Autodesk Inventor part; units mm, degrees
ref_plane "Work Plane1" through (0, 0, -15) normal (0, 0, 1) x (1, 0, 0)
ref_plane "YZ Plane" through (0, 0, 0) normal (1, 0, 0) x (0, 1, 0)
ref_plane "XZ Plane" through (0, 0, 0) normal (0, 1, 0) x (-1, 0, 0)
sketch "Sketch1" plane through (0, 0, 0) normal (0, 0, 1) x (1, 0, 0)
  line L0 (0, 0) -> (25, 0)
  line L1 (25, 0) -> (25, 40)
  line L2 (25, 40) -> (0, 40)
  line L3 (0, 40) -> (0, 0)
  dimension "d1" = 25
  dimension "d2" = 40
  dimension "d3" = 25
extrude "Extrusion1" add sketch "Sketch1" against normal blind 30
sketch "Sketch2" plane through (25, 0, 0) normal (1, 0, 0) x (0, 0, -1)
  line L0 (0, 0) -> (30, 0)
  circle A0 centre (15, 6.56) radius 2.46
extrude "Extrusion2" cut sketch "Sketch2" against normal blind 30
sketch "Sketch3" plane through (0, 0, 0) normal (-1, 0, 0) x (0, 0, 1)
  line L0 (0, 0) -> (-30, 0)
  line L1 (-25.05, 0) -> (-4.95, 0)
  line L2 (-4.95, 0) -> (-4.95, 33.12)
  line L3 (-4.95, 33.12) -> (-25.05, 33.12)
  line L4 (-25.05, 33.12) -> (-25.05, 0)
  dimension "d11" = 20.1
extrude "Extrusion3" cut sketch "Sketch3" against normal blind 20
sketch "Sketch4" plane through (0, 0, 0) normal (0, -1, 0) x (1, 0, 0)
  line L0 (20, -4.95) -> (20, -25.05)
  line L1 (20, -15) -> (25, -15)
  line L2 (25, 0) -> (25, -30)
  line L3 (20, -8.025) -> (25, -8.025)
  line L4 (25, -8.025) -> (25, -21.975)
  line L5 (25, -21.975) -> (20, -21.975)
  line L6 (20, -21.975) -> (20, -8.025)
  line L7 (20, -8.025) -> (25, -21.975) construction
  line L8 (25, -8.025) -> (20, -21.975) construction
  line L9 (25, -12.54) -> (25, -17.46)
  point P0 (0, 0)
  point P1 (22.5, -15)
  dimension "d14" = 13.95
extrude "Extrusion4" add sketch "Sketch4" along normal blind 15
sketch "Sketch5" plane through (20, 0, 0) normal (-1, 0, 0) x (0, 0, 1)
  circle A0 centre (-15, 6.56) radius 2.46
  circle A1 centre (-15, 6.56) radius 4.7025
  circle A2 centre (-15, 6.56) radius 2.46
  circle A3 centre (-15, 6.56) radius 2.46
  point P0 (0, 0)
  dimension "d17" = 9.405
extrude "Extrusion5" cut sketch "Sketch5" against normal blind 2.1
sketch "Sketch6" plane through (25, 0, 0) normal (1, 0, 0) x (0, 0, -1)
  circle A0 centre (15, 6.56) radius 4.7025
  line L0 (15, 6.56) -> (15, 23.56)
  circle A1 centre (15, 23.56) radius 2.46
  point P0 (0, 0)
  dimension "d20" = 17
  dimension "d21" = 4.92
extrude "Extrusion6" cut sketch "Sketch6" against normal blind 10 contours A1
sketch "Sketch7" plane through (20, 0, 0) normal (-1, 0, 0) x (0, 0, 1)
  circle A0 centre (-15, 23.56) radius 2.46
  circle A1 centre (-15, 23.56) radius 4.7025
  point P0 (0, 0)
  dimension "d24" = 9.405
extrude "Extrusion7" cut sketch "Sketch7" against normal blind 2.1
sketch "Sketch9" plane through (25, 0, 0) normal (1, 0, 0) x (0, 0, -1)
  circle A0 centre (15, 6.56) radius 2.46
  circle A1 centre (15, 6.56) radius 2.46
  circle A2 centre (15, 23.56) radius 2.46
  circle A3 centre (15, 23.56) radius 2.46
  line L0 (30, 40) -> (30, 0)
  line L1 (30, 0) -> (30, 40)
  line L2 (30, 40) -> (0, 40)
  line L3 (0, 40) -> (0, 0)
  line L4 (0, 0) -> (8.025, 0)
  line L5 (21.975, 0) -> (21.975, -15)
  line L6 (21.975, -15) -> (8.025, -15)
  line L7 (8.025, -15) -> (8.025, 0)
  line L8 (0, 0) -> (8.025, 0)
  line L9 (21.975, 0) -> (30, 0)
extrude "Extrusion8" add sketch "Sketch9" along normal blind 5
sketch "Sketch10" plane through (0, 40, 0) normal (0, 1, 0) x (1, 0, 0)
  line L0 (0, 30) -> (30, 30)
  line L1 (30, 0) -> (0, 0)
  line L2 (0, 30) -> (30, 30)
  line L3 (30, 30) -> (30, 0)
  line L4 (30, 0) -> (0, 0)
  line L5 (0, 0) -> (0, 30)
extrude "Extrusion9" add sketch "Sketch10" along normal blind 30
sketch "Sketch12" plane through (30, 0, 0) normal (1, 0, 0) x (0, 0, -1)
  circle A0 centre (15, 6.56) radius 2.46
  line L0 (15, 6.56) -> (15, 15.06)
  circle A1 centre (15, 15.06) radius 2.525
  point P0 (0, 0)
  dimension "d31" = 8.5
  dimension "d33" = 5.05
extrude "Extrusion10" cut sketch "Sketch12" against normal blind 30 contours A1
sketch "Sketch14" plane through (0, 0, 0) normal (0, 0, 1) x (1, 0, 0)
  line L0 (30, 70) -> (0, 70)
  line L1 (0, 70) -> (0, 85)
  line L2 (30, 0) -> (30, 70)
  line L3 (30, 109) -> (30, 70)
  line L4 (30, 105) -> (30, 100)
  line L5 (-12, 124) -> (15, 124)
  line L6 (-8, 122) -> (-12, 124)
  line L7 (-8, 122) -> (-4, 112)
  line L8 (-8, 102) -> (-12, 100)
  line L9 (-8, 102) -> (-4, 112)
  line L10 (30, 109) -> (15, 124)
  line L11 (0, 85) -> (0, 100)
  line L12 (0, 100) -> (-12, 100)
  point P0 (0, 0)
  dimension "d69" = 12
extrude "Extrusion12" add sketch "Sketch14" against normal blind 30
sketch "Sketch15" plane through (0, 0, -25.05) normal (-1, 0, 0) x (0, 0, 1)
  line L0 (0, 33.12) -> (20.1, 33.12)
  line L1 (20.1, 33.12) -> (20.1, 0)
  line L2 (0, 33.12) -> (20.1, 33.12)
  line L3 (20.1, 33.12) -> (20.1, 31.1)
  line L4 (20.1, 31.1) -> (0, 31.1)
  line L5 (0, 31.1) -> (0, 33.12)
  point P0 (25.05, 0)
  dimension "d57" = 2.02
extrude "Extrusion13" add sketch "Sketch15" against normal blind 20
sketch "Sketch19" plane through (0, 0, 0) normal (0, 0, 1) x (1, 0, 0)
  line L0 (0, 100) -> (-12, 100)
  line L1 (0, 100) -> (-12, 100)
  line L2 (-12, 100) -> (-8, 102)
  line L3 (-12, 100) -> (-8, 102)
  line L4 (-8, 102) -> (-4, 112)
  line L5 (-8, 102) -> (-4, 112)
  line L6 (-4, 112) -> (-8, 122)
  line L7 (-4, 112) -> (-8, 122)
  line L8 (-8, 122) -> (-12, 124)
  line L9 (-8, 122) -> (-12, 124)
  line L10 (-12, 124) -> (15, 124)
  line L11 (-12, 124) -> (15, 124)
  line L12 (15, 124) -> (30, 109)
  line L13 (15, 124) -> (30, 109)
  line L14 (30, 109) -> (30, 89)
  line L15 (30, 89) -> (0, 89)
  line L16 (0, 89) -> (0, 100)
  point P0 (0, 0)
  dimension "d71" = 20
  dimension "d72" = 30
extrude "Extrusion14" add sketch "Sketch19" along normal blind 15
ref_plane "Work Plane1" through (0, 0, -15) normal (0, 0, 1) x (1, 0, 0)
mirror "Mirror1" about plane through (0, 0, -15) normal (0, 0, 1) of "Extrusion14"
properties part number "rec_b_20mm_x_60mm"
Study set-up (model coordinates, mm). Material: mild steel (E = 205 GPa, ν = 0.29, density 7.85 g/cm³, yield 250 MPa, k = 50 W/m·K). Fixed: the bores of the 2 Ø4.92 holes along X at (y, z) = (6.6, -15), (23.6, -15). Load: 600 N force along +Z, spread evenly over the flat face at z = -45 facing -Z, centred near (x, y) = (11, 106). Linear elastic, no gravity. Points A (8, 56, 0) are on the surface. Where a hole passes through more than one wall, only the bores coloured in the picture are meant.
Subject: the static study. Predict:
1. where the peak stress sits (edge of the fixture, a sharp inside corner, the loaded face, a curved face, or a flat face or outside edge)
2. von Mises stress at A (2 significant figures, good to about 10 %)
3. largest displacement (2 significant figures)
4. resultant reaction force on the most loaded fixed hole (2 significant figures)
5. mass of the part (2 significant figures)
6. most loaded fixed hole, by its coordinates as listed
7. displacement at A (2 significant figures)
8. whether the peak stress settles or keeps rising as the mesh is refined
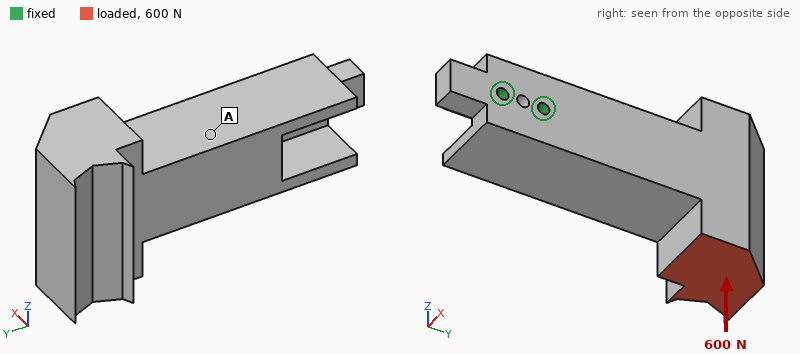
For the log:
edge of the fixture
6.4 MPa
38 µm
2.7 kN
1.1 kg
(23.6, -15)
11 µm
keeps rising
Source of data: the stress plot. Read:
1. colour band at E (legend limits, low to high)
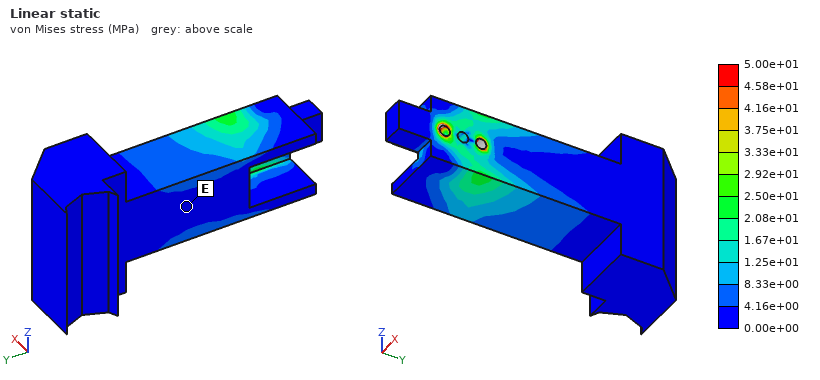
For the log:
0.00e+00 to 4.16e+00 MPa
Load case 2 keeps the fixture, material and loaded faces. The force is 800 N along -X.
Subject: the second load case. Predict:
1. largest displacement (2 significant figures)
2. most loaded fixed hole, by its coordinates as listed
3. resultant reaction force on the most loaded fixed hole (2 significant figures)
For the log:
83 µm
(23.6, -15)
3.4 kN
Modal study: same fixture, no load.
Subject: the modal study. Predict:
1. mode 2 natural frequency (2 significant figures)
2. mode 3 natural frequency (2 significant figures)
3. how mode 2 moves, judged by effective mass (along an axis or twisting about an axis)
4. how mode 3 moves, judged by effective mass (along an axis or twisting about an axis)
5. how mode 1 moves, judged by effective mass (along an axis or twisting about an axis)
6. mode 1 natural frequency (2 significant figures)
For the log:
920 Hz
2100 Hz
along Z
twisting about Y
along X
800 Hz
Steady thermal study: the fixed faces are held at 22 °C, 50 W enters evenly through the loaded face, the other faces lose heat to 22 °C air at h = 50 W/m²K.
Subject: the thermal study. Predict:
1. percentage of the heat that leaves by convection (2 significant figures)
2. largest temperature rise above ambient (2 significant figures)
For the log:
67 %
68 K
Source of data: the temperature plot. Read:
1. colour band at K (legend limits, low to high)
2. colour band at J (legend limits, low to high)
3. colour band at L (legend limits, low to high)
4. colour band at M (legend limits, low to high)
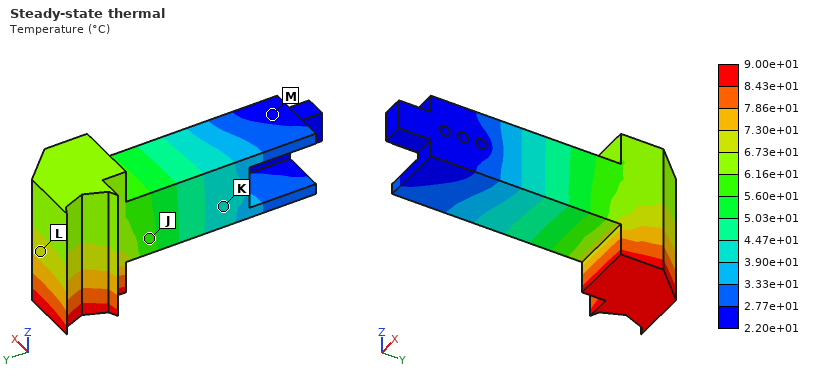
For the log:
3.90e+01 to 4.47e+01 °C
5.60e+01 to 6.16e+01 °C
6.73e+01 to 7.30e+01 °C
2.20e+01 to 2.77e+01 °C
